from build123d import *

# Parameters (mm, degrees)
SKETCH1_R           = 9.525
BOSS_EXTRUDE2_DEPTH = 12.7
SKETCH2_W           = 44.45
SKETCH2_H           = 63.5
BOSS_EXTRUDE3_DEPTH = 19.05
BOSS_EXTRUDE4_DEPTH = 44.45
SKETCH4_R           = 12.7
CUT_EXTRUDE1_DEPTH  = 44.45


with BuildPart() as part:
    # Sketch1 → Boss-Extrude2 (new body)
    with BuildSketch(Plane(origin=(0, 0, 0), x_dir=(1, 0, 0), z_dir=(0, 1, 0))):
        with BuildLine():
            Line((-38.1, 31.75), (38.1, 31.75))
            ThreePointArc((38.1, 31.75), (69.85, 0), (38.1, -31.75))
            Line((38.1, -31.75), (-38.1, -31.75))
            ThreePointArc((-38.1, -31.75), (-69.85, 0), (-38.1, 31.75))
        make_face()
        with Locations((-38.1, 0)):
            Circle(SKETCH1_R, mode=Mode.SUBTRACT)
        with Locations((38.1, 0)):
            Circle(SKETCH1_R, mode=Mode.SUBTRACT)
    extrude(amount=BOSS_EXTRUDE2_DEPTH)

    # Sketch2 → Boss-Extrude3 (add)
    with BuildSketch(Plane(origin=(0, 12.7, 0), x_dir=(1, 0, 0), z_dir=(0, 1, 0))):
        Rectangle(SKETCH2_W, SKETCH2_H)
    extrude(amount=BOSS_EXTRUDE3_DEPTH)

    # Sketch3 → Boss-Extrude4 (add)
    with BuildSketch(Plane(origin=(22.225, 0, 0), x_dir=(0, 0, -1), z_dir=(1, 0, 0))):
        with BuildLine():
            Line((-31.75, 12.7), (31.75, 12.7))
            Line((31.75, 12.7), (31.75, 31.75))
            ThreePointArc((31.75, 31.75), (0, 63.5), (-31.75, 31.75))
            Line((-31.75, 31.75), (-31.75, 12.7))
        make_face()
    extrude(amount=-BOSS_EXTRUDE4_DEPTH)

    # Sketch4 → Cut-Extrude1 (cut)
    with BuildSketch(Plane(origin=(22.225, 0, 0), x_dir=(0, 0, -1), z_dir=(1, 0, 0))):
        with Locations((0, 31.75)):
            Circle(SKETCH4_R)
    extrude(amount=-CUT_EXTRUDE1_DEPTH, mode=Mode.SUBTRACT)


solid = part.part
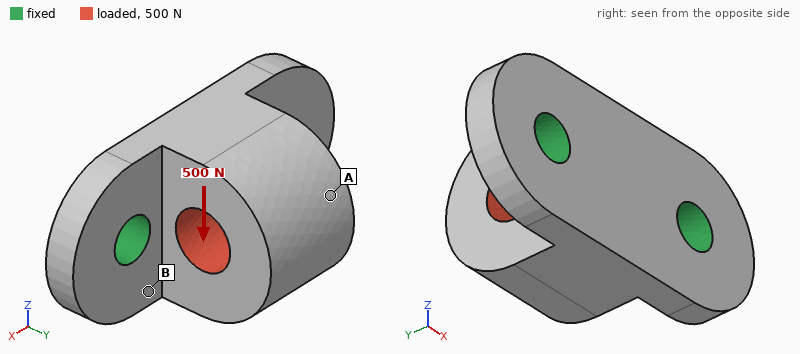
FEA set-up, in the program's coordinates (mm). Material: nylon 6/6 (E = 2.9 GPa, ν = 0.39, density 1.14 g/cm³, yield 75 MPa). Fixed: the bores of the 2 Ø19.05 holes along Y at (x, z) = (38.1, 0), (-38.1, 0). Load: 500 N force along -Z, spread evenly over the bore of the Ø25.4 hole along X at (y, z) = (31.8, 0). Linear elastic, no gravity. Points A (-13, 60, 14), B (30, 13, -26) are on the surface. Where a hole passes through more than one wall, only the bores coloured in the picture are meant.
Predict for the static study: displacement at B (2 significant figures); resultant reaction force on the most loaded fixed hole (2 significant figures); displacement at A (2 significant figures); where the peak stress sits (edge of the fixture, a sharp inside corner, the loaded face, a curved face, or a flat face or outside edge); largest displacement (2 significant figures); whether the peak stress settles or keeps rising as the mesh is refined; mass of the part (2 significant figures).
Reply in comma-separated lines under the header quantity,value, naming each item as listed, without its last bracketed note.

quantity,value
displacement at B,0.028 mm
resultant reaction force on the most loaded fixed hole,250 N
displacement at A,0.10 mm
where the peak stress sits,edge of the fixture
largest displacement,0.11 mm
whether the peak stress settles or keeps rising as the mesh is refined,keeps rising
mass of the part,220 g
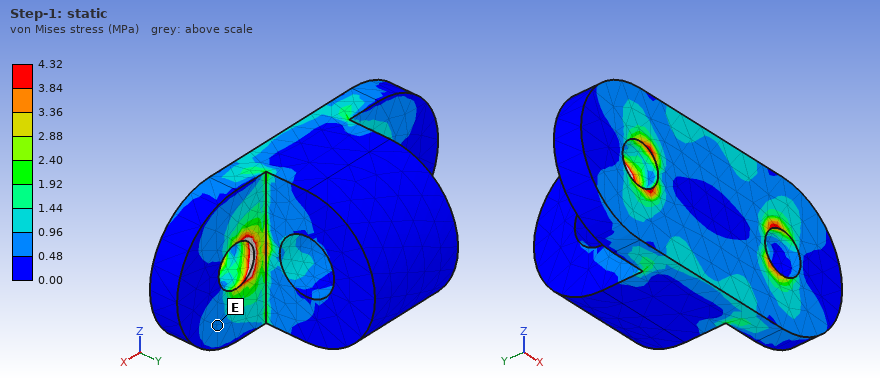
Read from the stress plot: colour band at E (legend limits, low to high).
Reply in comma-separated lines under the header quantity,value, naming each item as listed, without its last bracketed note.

quantity,value
colour band at E,0.48 to 0.96 MPa
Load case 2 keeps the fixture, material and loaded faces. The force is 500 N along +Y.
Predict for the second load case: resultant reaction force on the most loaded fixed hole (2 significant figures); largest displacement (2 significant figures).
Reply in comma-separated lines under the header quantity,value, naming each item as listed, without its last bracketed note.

quantity,value
resultant reaction force on the most loaded fixed hole,270 N
largest displacement,17 µm
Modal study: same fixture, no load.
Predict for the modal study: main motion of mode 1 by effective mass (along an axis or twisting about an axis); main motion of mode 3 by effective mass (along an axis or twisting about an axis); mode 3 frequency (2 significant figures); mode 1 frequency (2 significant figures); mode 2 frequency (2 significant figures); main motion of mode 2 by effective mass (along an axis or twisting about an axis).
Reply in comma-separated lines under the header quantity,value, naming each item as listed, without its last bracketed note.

quantity,value
main motion of mode 1 by effective mass,along Z
main motion of mode 3 by effective mass,along Y
mode 3 frequency,2300 Hz
mode 1 frequency,1000 Hz
mode 2 frequency,1800 Hz
main motion of mode 2 by effective mass,along X
